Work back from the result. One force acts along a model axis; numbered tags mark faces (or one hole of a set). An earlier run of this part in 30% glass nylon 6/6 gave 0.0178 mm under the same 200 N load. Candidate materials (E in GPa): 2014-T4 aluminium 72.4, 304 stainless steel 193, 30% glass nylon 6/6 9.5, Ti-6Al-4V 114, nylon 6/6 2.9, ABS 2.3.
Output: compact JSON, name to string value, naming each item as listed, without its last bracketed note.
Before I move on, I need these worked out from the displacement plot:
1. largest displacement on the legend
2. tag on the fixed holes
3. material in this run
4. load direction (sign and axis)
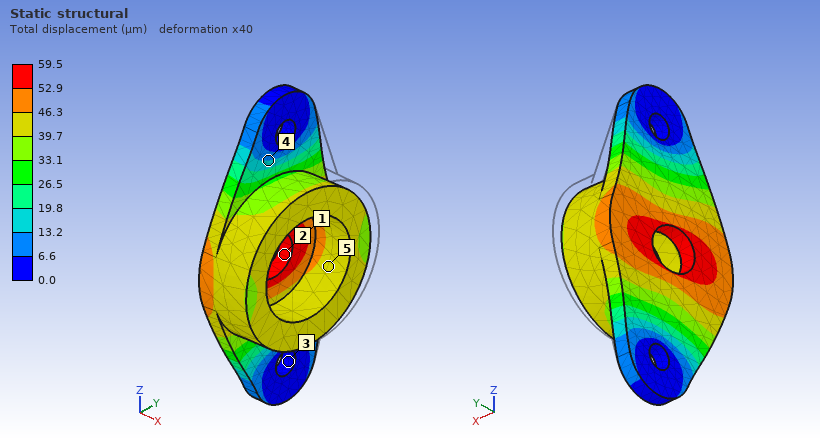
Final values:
{"largest displacement on the legend": "59.5 µm", "tag on the fixed holes": "3", "material in this run": "nylon 6/6", "load direction": "-Y"}
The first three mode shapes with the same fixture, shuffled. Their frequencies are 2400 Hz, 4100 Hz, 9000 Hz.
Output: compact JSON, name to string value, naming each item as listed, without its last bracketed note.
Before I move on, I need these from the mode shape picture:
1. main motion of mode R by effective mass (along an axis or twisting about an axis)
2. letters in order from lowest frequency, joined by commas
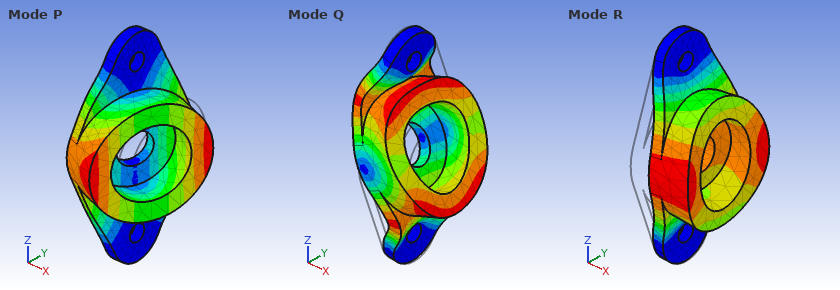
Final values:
{"main motion of mode R by effective mass": "along X", "letters in order from lowest frequency, joined by commas": "P, R, Q"}
